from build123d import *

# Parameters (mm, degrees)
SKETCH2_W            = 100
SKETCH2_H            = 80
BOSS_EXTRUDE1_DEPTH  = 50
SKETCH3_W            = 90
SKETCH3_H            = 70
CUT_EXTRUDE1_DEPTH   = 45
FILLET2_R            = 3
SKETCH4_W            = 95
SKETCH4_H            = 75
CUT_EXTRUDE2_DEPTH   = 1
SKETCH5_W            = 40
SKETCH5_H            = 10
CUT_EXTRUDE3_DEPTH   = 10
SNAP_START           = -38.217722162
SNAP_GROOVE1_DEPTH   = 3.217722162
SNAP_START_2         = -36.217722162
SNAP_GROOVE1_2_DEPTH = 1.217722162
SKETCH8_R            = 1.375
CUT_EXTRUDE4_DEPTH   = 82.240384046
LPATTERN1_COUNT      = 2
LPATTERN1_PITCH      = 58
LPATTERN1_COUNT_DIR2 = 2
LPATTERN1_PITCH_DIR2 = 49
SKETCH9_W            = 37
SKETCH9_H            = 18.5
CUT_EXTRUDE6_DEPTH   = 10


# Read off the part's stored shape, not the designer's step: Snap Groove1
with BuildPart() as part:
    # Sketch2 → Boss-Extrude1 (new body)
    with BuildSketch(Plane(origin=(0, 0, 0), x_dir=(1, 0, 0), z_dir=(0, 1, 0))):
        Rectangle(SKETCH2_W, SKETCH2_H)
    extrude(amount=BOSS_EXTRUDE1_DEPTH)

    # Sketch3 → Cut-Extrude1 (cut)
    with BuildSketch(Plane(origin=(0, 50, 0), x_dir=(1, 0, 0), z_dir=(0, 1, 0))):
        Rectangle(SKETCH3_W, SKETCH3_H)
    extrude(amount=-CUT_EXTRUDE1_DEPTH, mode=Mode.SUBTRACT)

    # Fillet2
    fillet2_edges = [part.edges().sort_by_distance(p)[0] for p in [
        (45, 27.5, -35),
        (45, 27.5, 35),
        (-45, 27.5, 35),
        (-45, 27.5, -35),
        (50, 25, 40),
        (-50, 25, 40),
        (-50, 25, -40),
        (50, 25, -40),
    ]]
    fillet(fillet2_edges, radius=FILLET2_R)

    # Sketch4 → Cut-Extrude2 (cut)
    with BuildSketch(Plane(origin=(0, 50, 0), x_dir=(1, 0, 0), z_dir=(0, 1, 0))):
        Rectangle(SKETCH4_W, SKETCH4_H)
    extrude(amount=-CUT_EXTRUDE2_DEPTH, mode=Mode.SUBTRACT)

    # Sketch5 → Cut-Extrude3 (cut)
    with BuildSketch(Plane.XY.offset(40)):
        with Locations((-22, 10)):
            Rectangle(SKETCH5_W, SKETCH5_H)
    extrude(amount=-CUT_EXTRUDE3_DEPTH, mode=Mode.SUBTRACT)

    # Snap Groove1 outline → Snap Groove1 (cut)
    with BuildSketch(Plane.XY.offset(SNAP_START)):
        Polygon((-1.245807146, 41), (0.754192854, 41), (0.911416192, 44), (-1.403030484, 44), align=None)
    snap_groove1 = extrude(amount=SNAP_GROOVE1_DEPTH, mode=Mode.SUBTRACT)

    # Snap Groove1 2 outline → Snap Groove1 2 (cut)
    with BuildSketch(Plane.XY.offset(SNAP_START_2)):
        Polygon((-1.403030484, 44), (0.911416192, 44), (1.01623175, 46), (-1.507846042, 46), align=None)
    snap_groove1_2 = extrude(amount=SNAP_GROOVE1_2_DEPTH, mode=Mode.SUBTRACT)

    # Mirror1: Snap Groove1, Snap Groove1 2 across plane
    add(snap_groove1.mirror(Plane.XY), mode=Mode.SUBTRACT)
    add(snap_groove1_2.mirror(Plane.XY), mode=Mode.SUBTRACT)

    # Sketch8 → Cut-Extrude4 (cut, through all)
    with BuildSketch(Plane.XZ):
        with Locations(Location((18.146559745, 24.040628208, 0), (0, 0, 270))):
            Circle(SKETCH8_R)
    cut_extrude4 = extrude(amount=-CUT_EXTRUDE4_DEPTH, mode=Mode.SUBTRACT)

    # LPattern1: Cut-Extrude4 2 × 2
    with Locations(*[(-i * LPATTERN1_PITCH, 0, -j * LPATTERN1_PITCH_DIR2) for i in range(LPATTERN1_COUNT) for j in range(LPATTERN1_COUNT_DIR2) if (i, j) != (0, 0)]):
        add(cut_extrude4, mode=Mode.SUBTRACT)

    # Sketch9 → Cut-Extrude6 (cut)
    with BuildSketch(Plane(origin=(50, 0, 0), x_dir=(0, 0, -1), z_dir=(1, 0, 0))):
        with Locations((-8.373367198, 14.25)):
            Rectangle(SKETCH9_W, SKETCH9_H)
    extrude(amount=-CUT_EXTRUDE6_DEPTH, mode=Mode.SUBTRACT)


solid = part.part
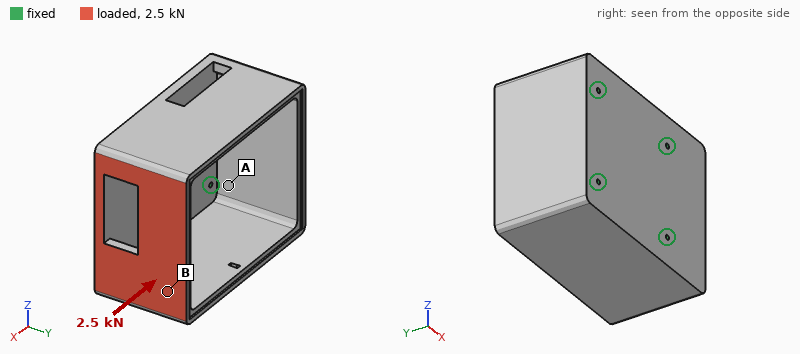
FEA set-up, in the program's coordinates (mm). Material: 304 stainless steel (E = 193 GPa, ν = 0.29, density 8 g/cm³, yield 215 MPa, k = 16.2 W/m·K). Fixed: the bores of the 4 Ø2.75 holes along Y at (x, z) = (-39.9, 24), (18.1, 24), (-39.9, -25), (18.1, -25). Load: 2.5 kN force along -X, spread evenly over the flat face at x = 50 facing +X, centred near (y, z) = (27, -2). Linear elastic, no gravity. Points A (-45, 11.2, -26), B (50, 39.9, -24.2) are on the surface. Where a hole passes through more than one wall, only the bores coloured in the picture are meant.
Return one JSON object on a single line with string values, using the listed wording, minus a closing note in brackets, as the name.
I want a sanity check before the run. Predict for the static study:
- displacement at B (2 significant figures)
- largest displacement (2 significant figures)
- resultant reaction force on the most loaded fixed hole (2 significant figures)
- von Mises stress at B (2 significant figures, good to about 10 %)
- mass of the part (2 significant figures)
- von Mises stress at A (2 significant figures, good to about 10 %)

{"displacement at B": "30 µm", "largest displacement": "66 µm", "resultant reaction force on the most loaded fixed hole": "980 N", "von Mises stress at B": "23 MPa", "mass of the part": "880 g", "von Mises stress at A": "7.4 MPa"}
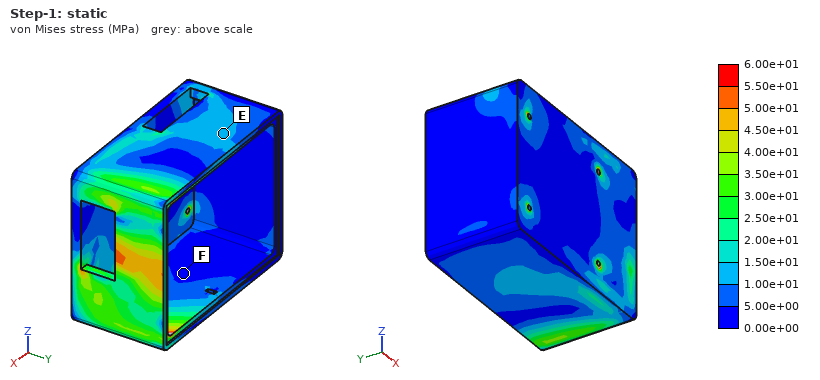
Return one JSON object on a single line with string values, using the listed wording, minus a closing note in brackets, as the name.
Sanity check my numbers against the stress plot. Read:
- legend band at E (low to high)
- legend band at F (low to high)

{"legend band at E": "1.00e+01 to 1.50e+01 MPa", "legend band at F": "0.00e+00 to 5.00e+00 MPa"}
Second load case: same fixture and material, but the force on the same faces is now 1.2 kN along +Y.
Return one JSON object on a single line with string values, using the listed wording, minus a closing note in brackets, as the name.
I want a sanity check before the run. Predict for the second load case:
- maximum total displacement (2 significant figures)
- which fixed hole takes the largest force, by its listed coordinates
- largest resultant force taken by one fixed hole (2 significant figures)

{"maximum total displacement": "20 µm", "which fixed hole takes the largest force, by its listed coordinates": "(18.1, -25)", "largest resultant force taken by one fixed hole": "970 N"}
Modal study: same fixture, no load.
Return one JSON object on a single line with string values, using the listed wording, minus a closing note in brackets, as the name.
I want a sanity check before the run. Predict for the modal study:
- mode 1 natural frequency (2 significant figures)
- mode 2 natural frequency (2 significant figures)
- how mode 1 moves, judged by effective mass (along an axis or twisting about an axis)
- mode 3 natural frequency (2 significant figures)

{"mode 1 natural frequency": "2000 Hz", "mode 2 natural frequency": "2500 Hz", "how mode 1 moves, judged by effective mass": "along Z", "mode 3 natural frequency": "2800 Hz"}
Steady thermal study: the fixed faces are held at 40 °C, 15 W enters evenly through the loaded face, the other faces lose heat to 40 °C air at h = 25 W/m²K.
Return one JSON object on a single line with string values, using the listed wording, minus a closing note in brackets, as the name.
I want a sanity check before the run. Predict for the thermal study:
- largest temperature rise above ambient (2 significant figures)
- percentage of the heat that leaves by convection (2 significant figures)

{"largest temperature rise above ambient": "56 K", "percentage of the heat that leaves by convection": "73 %"}
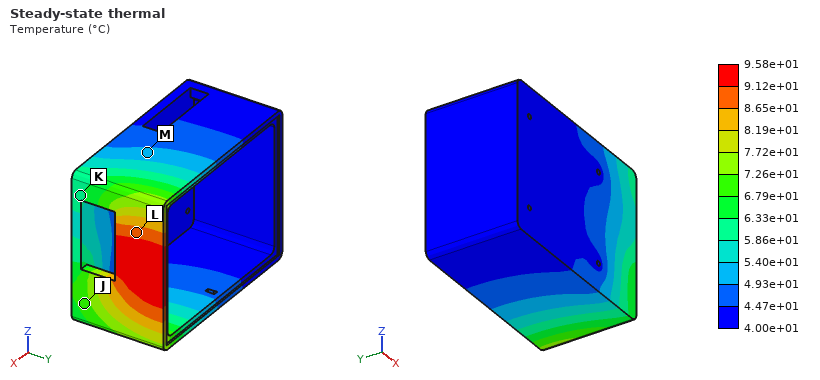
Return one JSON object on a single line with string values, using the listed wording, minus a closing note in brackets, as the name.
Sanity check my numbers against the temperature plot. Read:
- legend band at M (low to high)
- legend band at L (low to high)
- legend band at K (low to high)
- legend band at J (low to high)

{"legend band at M": "4.93e+01 to 5.40e+01 °C", "legend band at L": "8.65e+01 to 9.12e+01 °C", "legend band at K": "5.86e+01 to 6.33e+01 °C", "legend band at J": "6.79e+01 to 7.26e+01 °C"}
